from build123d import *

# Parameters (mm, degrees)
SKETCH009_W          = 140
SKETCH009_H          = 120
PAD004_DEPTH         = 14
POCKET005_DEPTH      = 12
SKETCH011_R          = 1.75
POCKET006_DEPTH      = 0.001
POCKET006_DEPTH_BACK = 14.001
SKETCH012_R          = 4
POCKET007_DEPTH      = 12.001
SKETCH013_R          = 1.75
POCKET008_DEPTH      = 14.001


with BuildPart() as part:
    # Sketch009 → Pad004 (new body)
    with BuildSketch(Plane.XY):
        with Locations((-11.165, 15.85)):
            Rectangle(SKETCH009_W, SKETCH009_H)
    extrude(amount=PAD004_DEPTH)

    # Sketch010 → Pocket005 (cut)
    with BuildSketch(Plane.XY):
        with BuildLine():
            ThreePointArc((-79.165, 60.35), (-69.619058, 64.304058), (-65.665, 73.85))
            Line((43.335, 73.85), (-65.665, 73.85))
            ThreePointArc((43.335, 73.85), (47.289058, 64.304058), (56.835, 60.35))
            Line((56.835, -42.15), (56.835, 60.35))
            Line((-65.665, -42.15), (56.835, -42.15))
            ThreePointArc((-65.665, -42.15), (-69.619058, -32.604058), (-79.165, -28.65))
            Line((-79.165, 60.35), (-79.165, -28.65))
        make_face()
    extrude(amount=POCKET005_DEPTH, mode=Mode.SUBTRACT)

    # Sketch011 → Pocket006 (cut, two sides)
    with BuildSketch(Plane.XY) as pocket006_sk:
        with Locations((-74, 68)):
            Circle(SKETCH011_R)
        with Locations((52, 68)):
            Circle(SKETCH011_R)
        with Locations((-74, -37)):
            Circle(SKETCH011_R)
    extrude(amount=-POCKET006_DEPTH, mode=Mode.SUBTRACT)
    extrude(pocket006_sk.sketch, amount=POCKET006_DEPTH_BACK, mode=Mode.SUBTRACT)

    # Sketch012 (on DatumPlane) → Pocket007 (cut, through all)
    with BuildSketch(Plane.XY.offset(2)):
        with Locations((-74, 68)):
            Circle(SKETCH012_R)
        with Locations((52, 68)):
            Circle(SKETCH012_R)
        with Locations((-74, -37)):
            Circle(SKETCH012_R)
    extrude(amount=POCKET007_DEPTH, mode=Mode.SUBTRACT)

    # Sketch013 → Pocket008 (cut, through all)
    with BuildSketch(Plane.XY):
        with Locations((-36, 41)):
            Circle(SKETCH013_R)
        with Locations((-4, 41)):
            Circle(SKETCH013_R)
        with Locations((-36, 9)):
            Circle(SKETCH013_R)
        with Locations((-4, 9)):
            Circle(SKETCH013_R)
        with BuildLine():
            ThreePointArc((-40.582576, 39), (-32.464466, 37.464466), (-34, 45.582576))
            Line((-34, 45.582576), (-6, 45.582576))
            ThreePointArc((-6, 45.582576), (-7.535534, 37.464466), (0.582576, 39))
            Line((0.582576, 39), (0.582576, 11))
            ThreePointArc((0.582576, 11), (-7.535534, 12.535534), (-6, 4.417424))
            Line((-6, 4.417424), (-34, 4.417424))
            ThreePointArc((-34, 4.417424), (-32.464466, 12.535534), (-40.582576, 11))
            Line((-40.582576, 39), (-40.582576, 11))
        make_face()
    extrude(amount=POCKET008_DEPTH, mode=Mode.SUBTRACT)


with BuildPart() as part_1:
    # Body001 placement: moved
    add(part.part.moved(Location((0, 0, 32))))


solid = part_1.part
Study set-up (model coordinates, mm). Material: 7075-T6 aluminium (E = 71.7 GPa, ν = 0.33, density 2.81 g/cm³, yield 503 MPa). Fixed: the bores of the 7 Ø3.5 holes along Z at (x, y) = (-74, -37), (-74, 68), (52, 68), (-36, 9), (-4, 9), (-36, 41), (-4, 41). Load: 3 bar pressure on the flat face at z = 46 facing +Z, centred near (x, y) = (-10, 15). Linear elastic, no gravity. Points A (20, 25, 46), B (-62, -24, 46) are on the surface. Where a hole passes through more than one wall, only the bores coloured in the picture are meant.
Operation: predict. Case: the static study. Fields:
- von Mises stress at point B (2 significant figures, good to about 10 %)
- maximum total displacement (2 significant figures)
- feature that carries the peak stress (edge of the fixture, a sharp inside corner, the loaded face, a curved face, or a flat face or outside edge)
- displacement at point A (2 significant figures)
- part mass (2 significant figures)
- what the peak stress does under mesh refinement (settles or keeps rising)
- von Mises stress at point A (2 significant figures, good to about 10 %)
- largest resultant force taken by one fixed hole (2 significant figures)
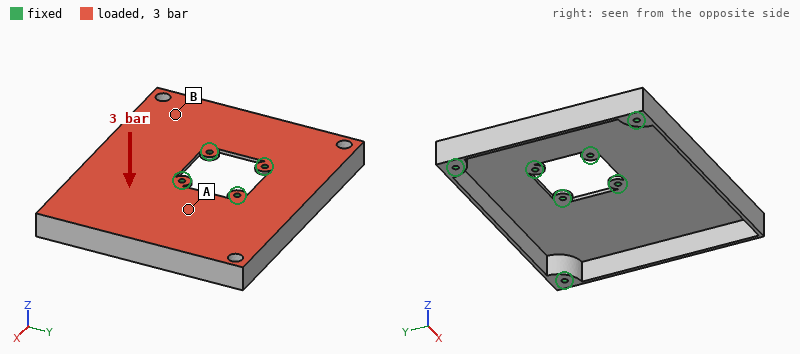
31 MPa
1.8 mm
edge of the fixture
0.49 mm
130 g
keeps rising
90 MPa
3.4 kN
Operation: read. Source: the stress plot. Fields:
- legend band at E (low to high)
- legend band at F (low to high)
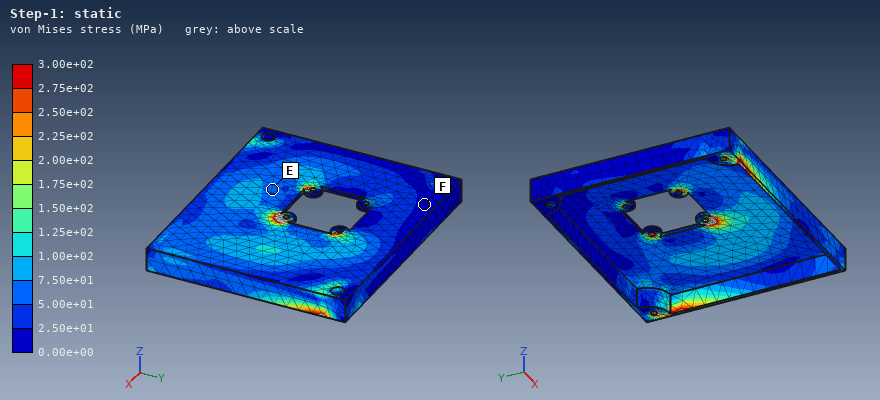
5.00e+01 to 7.50e+01 MPa
0.00e+00 to 2.50e+01 MPa
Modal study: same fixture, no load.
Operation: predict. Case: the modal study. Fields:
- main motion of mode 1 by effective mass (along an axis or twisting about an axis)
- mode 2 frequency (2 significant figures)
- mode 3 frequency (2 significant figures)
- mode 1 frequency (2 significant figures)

along Z
2200 Hz
2400 Hz
910 Hz
